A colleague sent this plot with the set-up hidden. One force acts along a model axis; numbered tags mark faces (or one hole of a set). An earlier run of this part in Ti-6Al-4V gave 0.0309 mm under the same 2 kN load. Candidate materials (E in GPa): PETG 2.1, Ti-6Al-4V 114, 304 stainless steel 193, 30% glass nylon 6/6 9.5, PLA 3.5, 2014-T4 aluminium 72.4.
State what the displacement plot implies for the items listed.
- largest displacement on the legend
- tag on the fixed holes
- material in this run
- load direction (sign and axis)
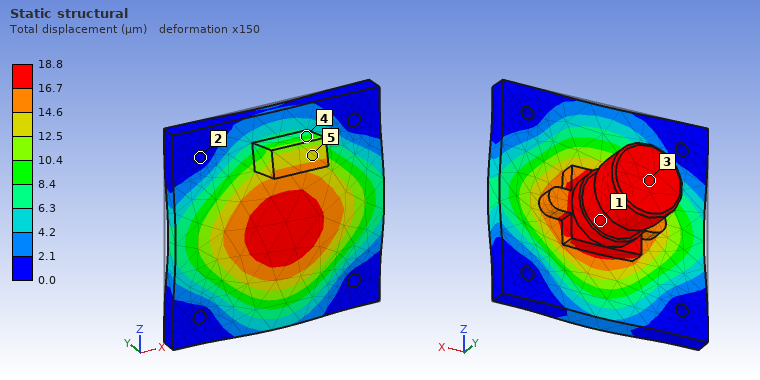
18.8 µm
2
304 stainless steel
-Y
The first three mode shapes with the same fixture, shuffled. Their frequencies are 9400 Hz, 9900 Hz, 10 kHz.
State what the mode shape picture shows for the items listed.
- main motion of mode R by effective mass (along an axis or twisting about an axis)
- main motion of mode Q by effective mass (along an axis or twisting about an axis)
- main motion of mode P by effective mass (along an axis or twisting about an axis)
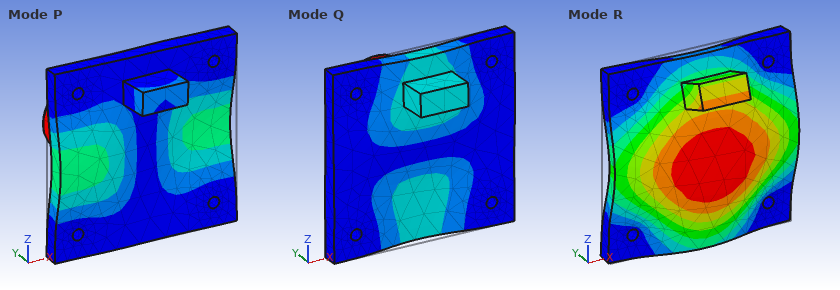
along Y
along Z
along X
